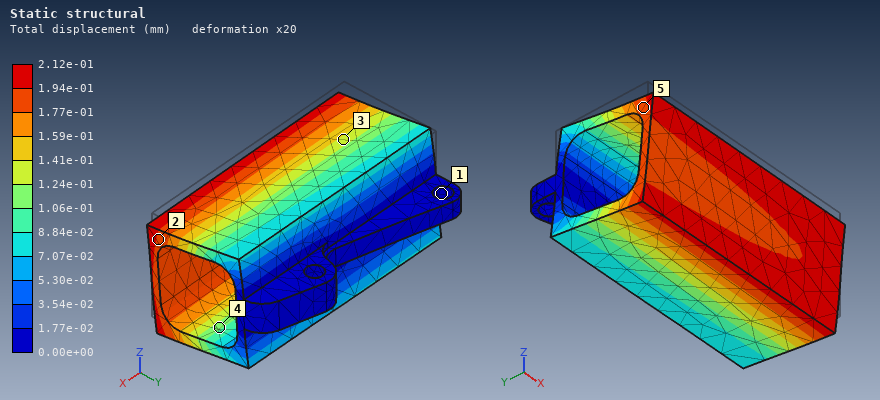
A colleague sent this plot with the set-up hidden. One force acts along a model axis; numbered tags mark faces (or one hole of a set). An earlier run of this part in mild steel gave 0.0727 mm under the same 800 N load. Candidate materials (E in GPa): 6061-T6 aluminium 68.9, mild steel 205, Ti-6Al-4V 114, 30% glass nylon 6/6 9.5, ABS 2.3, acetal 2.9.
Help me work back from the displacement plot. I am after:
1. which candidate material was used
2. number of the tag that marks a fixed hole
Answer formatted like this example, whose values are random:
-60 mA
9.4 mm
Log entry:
6061-T6 aluminium
1
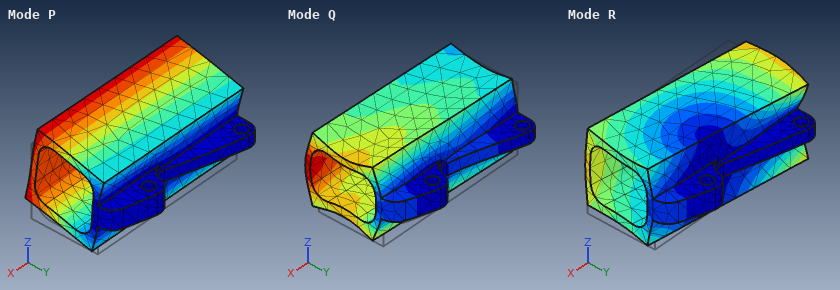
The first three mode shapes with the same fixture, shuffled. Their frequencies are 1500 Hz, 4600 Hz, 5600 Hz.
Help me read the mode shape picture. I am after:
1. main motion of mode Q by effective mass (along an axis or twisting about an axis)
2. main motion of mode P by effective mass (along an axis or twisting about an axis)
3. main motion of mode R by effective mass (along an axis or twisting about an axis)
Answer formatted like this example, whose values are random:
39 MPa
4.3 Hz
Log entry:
along Y
along Z
along X
